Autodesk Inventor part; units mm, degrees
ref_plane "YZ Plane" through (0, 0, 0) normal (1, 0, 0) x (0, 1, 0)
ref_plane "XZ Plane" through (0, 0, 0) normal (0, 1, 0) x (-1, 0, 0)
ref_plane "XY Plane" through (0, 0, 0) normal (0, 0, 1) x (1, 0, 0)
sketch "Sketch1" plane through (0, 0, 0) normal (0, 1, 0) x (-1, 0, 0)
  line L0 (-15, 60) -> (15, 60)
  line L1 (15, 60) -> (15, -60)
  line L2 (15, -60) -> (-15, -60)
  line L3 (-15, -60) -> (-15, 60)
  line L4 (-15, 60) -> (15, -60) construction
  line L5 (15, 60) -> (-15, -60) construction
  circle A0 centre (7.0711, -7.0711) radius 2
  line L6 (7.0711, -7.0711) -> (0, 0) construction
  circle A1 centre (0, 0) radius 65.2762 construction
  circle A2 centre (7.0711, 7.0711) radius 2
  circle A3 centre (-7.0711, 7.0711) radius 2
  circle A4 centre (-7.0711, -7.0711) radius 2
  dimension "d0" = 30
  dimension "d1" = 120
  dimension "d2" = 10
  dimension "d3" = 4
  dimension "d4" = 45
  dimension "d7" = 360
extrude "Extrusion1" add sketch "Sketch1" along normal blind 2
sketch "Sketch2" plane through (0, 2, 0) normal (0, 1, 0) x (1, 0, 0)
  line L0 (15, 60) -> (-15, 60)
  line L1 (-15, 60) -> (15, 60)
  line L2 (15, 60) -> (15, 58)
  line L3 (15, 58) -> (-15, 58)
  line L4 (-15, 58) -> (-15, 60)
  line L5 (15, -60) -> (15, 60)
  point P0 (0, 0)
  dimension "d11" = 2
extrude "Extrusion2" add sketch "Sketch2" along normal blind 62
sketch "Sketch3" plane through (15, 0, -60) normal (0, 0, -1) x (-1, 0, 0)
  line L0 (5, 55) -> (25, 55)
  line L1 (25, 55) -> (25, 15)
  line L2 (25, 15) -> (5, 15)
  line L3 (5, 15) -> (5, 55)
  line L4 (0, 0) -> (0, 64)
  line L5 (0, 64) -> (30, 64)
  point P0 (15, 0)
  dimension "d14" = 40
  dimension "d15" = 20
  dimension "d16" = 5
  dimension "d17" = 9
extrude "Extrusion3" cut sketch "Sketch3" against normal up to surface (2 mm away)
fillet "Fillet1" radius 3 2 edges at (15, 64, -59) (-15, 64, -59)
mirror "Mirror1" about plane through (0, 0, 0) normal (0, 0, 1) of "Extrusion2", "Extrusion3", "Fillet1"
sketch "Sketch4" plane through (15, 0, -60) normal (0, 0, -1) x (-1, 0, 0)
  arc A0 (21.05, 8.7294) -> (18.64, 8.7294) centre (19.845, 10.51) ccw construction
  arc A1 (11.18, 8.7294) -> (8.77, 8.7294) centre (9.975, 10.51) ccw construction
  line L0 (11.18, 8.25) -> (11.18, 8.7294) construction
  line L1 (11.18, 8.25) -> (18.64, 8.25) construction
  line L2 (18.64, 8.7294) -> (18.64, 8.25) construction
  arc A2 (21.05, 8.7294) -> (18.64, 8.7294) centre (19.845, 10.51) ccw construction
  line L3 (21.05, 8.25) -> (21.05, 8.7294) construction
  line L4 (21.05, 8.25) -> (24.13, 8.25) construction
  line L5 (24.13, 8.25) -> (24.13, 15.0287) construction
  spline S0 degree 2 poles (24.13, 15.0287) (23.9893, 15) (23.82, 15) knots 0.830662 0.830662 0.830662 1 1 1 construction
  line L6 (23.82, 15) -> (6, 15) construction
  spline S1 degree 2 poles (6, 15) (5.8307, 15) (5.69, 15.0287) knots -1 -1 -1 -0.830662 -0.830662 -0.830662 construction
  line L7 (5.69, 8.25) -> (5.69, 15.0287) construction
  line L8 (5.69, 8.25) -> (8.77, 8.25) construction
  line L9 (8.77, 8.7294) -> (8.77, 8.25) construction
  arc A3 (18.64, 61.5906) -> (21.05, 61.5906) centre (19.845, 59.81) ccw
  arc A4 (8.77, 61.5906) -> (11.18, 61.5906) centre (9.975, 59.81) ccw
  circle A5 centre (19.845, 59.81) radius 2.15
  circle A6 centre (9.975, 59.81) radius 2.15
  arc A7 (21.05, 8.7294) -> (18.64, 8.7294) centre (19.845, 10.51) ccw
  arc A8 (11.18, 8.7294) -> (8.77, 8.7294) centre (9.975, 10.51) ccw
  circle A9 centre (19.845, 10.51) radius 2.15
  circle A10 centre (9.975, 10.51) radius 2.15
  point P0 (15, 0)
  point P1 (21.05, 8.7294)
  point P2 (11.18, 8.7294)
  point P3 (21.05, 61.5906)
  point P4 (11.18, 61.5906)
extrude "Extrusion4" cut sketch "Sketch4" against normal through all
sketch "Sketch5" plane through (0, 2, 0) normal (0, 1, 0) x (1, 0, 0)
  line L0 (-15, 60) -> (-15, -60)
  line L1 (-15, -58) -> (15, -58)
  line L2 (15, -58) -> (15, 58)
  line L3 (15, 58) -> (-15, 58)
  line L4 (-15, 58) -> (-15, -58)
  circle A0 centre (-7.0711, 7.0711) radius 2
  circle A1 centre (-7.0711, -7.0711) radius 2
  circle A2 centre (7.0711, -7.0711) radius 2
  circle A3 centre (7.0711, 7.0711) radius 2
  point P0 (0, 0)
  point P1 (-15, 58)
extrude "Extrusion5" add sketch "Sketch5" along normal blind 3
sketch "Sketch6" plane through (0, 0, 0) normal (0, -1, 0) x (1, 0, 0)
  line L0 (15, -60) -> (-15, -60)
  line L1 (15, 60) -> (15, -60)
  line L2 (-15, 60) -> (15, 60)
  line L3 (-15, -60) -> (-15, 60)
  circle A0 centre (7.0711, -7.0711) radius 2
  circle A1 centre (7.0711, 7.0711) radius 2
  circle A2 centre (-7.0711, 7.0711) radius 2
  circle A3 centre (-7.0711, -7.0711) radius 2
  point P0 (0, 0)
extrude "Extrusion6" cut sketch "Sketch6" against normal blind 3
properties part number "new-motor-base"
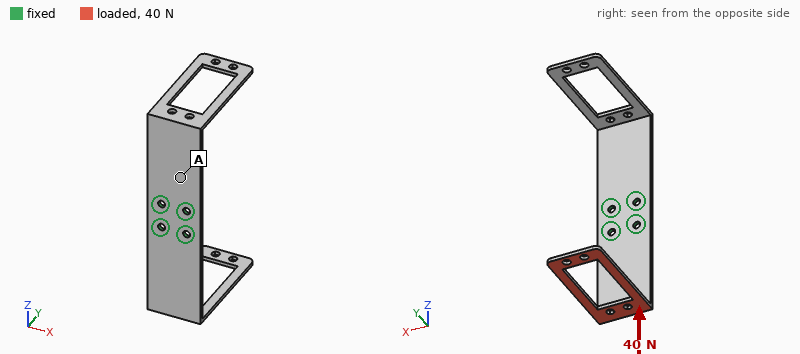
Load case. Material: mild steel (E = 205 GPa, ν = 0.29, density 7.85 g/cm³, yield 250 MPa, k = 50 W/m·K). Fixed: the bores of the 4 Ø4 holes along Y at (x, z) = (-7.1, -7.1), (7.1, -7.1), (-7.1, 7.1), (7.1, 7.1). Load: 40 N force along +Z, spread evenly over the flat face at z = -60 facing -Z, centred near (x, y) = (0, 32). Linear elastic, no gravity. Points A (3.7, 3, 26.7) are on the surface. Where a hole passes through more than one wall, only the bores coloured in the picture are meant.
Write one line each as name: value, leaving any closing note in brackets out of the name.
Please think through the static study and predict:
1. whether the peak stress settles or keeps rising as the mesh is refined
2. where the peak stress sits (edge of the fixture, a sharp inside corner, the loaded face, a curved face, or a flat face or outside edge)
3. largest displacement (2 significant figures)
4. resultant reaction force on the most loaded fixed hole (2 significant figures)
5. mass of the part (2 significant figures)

whether the peak stress settles or keeps rising as the mesh is refined: keeps rising
where the peak stress sits: a sharp inside corner
largest displacement: 1.4 mm
resultant reaction force on the most loaded fixed hole: 18 N
mass of the part: 84 g
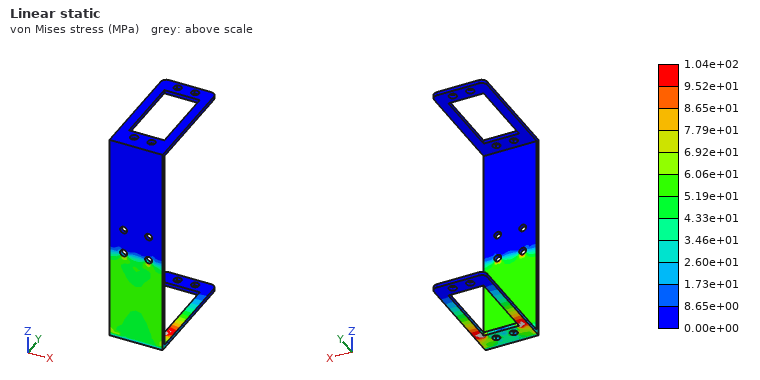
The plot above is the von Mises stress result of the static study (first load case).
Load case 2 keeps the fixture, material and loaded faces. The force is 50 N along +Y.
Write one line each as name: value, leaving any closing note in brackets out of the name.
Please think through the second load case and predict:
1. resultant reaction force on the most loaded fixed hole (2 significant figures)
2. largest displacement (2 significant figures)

resultant reaction force on the most loaded fixed hole: 35 N
largest displacement: 1.1 mm
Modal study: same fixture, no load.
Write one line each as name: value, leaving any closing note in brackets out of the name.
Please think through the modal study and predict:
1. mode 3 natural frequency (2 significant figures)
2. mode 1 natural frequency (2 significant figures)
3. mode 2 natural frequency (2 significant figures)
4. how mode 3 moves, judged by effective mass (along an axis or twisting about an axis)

mode 3 natural frequency: 420 Hz
mode 1 natural frequency: 230 Hz
mode 2 natural frequency: 230 Hz
how mode 3 moves, judged by effective mass: along X
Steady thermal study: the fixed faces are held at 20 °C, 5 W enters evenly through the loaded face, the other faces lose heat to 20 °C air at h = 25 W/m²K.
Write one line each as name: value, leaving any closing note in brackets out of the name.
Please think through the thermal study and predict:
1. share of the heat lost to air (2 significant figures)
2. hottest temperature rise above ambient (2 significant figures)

share of the heat lost to air: 70 %
hottest temperature rise above ambient: 78 K
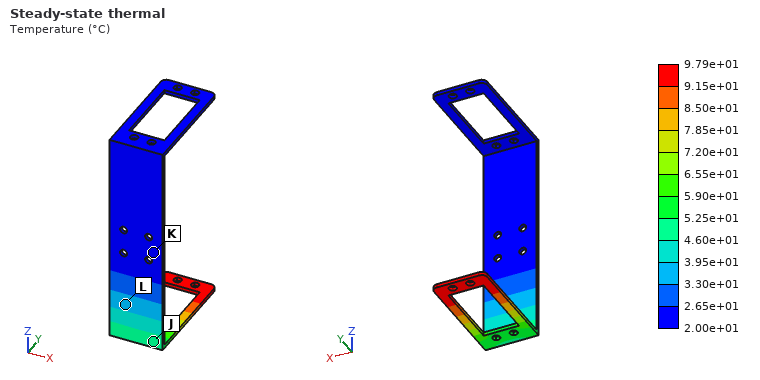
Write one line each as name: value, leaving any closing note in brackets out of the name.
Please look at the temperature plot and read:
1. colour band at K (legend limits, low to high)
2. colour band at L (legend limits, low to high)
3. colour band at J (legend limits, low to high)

colour band at K: 2.00e+01 to 2.65e+01 °C
colour band at L: 3.30e+01 to 3.95e+01 °C
colour band at J: 4.60e+01 to 5.25e+01 °C
